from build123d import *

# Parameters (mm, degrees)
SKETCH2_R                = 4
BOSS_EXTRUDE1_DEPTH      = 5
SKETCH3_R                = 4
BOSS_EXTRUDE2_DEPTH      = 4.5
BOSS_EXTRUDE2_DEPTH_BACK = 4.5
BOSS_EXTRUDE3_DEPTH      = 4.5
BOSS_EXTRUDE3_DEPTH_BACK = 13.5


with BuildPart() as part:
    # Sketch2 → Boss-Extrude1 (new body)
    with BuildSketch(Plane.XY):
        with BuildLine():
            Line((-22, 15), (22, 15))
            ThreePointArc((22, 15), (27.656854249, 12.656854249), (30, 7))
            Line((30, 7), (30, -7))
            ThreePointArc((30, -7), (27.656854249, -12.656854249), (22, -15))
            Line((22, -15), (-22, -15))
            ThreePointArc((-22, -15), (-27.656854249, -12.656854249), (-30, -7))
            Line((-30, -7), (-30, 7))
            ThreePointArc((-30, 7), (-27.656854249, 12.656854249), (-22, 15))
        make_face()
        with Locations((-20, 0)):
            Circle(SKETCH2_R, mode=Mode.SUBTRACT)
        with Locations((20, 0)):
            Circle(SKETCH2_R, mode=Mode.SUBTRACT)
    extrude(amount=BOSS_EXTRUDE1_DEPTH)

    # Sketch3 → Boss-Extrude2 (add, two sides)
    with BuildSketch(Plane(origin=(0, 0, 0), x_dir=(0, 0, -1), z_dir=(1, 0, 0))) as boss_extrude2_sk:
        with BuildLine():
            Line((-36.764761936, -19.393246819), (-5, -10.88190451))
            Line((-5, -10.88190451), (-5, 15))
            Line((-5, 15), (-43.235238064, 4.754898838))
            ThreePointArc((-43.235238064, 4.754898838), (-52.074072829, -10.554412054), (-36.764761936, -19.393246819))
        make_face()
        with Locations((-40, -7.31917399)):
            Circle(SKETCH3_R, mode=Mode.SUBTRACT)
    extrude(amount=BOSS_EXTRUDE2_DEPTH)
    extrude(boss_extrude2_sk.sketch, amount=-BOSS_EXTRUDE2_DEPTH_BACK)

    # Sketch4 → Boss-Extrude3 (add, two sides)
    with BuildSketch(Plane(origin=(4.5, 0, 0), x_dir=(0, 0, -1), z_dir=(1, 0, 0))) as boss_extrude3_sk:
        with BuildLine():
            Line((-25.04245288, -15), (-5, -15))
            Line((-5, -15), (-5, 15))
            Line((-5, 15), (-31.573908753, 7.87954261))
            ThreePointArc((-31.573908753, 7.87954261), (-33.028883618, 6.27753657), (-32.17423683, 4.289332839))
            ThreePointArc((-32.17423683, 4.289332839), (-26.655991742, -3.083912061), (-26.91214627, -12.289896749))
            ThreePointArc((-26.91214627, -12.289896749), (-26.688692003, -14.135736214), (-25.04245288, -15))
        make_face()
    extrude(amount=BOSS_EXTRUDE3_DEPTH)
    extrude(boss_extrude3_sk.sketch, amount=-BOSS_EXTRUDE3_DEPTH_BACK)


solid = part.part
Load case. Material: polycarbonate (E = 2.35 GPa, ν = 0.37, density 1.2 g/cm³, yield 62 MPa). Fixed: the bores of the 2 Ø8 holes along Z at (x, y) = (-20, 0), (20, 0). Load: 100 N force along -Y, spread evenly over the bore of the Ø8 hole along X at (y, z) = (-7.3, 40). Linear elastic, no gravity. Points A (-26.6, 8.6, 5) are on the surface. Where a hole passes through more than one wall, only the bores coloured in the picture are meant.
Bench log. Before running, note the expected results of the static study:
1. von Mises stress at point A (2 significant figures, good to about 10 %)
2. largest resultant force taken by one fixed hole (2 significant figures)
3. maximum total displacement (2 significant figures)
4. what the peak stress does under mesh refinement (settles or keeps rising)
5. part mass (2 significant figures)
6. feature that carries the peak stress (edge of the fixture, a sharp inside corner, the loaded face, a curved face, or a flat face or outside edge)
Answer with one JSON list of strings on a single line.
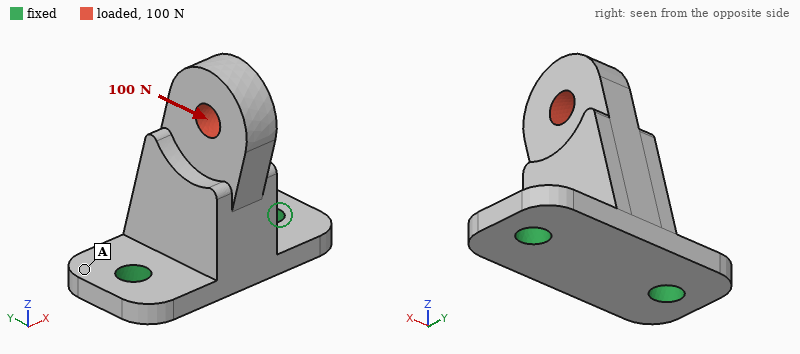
["3.1 MPa", "50 N", "0.68 mm", "keeps rising", "29 g", "edge of the fixture"]
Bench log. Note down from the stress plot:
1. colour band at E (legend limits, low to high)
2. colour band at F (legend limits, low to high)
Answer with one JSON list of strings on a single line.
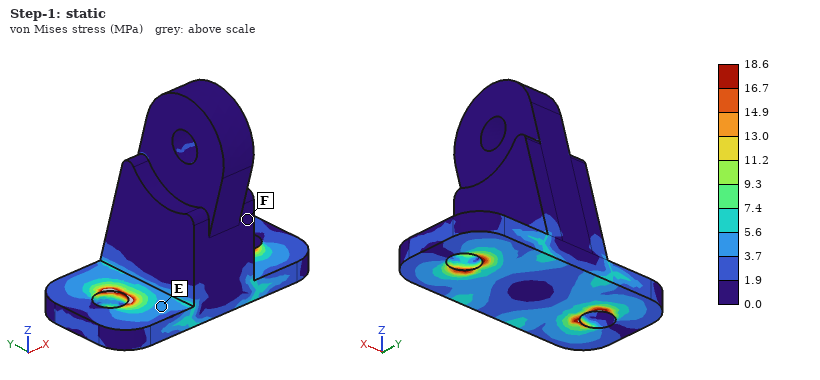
["3.7 to 5.6 MPa", "0.0 to 1.9 MPa"]
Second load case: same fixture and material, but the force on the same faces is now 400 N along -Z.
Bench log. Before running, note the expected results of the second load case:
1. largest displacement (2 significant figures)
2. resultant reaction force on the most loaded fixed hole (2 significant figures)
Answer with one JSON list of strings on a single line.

["0.55 mm", "210 N"]
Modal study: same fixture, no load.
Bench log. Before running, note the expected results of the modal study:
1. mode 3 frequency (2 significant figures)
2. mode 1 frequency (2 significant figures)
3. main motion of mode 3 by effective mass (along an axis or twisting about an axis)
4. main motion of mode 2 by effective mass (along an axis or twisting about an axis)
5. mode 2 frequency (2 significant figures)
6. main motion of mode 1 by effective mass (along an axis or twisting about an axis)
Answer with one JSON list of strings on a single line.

["2500 Hz", "760 Hz", "along Z", "along X", "1300 Hz", "along Y"]
